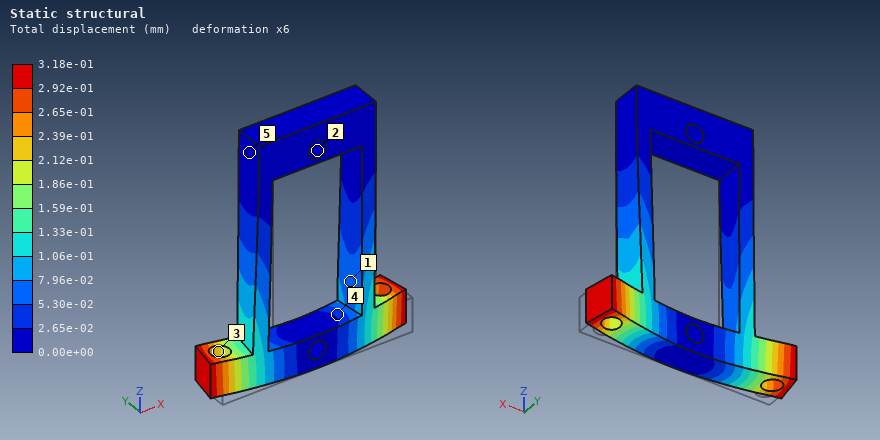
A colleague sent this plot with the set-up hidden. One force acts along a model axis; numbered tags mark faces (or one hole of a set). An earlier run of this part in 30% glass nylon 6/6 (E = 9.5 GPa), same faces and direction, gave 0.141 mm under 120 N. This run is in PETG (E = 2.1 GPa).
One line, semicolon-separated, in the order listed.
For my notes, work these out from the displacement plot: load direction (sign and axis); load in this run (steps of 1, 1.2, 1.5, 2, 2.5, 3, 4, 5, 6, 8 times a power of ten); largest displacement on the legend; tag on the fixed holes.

+Y; 60 N; 3.18e-01 mm; 2
